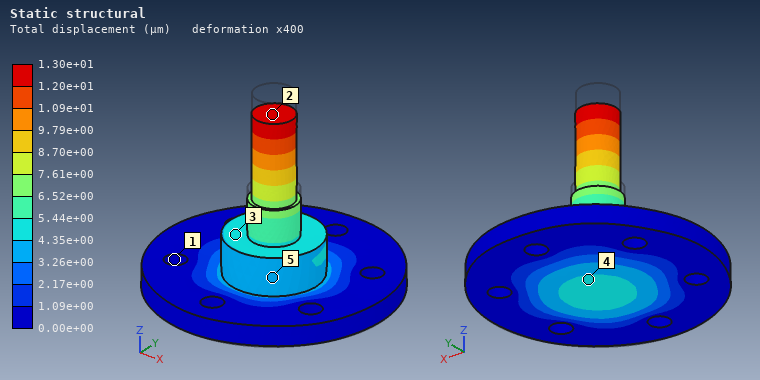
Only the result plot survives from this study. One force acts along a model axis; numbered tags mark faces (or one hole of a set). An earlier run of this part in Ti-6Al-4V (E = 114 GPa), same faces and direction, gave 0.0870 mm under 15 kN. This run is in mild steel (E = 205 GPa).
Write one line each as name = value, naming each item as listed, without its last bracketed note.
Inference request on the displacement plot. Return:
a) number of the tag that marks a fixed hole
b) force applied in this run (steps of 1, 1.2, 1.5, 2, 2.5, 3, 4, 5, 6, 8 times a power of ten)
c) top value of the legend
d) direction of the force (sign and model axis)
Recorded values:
number of the tag that marks a fixed hole = 1
force applied in this run = 4 kN
top value of the legend = 1.30e+01 µm
direction of the force = -Z
